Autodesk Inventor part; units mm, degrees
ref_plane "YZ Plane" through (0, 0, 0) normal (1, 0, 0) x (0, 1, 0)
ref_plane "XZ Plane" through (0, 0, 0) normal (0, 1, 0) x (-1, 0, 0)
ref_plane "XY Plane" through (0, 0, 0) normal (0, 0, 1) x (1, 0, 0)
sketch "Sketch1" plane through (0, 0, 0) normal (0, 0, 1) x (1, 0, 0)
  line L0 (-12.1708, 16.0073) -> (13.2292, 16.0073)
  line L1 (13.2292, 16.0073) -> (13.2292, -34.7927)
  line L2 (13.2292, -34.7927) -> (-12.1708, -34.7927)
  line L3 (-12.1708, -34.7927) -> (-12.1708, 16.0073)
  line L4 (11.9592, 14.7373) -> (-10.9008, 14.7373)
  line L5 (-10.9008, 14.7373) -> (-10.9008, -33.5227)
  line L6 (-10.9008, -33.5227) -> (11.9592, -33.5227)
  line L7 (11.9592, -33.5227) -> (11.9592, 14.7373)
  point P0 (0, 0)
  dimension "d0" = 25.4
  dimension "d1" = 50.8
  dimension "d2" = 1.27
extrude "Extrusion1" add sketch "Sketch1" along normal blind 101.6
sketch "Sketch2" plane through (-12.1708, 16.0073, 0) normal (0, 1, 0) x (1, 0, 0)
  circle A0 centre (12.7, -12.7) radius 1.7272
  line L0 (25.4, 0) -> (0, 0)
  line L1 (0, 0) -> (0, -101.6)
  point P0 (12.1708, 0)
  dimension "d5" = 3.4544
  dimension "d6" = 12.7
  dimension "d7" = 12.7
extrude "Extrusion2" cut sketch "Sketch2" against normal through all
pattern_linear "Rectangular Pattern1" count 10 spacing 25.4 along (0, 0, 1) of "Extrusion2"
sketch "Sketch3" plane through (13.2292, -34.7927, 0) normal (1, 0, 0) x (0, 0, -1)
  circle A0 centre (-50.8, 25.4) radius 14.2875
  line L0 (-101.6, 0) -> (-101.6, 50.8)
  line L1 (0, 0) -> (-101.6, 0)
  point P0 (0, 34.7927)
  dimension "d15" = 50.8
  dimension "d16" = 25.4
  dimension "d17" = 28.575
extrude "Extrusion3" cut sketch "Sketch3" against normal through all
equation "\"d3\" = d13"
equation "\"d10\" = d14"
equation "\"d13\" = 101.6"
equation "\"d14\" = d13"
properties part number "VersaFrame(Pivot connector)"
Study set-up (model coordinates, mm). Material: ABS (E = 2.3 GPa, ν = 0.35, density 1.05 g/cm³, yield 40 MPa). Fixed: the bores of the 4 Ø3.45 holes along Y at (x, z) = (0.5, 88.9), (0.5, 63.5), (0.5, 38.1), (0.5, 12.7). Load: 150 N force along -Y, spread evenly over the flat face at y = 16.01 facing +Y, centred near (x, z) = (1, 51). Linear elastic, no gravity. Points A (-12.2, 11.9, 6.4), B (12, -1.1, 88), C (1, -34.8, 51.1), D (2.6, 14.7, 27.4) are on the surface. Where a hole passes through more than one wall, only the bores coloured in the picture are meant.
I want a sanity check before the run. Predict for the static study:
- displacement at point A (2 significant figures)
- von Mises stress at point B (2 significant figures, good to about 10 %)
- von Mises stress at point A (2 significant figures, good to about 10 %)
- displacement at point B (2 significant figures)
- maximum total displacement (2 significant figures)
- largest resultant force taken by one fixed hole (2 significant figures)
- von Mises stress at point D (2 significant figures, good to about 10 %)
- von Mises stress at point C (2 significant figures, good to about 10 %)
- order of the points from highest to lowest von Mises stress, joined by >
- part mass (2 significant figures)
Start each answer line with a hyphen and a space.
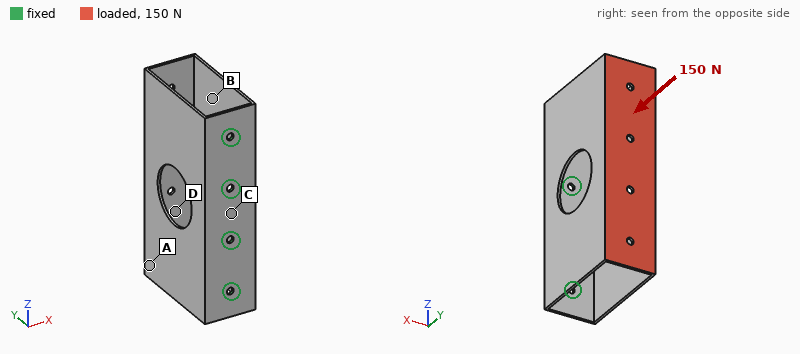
- 0.72 mm
- 4.2 MPa
- 2.2 MPa
- 1.1 mm
- 1.3 mm
- 39 N
- 12 MPa
- 15 MPa
- C > D > B > A
- 18 g
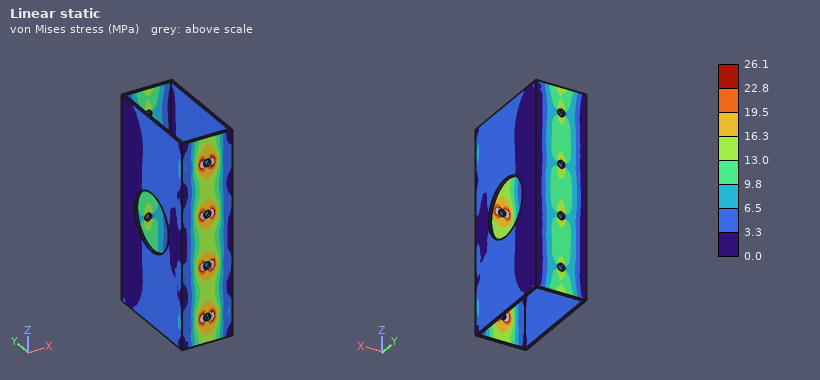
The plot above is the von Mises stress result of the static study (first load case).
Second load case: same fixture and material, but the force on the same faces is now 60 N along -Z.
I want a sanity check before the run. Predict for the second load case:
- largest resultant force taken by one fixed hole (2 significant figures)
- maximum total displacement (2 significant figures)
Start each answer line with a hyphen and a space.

- 37 N
- 1.1 mm
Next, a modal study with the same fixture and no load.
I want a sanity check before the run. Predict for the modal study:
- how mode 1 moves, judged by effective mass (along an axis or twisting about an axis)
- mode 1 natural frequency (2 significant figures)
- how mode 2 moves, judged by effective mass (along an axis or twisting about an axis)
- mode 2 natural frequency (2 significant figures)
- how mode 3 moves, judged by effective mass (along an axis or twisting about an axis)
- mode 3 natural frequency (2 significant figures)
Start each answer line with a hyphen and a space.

- along X
- 93 Hz
- twisting about Y
- 310 Hz
- along Z
- 380 Hz
